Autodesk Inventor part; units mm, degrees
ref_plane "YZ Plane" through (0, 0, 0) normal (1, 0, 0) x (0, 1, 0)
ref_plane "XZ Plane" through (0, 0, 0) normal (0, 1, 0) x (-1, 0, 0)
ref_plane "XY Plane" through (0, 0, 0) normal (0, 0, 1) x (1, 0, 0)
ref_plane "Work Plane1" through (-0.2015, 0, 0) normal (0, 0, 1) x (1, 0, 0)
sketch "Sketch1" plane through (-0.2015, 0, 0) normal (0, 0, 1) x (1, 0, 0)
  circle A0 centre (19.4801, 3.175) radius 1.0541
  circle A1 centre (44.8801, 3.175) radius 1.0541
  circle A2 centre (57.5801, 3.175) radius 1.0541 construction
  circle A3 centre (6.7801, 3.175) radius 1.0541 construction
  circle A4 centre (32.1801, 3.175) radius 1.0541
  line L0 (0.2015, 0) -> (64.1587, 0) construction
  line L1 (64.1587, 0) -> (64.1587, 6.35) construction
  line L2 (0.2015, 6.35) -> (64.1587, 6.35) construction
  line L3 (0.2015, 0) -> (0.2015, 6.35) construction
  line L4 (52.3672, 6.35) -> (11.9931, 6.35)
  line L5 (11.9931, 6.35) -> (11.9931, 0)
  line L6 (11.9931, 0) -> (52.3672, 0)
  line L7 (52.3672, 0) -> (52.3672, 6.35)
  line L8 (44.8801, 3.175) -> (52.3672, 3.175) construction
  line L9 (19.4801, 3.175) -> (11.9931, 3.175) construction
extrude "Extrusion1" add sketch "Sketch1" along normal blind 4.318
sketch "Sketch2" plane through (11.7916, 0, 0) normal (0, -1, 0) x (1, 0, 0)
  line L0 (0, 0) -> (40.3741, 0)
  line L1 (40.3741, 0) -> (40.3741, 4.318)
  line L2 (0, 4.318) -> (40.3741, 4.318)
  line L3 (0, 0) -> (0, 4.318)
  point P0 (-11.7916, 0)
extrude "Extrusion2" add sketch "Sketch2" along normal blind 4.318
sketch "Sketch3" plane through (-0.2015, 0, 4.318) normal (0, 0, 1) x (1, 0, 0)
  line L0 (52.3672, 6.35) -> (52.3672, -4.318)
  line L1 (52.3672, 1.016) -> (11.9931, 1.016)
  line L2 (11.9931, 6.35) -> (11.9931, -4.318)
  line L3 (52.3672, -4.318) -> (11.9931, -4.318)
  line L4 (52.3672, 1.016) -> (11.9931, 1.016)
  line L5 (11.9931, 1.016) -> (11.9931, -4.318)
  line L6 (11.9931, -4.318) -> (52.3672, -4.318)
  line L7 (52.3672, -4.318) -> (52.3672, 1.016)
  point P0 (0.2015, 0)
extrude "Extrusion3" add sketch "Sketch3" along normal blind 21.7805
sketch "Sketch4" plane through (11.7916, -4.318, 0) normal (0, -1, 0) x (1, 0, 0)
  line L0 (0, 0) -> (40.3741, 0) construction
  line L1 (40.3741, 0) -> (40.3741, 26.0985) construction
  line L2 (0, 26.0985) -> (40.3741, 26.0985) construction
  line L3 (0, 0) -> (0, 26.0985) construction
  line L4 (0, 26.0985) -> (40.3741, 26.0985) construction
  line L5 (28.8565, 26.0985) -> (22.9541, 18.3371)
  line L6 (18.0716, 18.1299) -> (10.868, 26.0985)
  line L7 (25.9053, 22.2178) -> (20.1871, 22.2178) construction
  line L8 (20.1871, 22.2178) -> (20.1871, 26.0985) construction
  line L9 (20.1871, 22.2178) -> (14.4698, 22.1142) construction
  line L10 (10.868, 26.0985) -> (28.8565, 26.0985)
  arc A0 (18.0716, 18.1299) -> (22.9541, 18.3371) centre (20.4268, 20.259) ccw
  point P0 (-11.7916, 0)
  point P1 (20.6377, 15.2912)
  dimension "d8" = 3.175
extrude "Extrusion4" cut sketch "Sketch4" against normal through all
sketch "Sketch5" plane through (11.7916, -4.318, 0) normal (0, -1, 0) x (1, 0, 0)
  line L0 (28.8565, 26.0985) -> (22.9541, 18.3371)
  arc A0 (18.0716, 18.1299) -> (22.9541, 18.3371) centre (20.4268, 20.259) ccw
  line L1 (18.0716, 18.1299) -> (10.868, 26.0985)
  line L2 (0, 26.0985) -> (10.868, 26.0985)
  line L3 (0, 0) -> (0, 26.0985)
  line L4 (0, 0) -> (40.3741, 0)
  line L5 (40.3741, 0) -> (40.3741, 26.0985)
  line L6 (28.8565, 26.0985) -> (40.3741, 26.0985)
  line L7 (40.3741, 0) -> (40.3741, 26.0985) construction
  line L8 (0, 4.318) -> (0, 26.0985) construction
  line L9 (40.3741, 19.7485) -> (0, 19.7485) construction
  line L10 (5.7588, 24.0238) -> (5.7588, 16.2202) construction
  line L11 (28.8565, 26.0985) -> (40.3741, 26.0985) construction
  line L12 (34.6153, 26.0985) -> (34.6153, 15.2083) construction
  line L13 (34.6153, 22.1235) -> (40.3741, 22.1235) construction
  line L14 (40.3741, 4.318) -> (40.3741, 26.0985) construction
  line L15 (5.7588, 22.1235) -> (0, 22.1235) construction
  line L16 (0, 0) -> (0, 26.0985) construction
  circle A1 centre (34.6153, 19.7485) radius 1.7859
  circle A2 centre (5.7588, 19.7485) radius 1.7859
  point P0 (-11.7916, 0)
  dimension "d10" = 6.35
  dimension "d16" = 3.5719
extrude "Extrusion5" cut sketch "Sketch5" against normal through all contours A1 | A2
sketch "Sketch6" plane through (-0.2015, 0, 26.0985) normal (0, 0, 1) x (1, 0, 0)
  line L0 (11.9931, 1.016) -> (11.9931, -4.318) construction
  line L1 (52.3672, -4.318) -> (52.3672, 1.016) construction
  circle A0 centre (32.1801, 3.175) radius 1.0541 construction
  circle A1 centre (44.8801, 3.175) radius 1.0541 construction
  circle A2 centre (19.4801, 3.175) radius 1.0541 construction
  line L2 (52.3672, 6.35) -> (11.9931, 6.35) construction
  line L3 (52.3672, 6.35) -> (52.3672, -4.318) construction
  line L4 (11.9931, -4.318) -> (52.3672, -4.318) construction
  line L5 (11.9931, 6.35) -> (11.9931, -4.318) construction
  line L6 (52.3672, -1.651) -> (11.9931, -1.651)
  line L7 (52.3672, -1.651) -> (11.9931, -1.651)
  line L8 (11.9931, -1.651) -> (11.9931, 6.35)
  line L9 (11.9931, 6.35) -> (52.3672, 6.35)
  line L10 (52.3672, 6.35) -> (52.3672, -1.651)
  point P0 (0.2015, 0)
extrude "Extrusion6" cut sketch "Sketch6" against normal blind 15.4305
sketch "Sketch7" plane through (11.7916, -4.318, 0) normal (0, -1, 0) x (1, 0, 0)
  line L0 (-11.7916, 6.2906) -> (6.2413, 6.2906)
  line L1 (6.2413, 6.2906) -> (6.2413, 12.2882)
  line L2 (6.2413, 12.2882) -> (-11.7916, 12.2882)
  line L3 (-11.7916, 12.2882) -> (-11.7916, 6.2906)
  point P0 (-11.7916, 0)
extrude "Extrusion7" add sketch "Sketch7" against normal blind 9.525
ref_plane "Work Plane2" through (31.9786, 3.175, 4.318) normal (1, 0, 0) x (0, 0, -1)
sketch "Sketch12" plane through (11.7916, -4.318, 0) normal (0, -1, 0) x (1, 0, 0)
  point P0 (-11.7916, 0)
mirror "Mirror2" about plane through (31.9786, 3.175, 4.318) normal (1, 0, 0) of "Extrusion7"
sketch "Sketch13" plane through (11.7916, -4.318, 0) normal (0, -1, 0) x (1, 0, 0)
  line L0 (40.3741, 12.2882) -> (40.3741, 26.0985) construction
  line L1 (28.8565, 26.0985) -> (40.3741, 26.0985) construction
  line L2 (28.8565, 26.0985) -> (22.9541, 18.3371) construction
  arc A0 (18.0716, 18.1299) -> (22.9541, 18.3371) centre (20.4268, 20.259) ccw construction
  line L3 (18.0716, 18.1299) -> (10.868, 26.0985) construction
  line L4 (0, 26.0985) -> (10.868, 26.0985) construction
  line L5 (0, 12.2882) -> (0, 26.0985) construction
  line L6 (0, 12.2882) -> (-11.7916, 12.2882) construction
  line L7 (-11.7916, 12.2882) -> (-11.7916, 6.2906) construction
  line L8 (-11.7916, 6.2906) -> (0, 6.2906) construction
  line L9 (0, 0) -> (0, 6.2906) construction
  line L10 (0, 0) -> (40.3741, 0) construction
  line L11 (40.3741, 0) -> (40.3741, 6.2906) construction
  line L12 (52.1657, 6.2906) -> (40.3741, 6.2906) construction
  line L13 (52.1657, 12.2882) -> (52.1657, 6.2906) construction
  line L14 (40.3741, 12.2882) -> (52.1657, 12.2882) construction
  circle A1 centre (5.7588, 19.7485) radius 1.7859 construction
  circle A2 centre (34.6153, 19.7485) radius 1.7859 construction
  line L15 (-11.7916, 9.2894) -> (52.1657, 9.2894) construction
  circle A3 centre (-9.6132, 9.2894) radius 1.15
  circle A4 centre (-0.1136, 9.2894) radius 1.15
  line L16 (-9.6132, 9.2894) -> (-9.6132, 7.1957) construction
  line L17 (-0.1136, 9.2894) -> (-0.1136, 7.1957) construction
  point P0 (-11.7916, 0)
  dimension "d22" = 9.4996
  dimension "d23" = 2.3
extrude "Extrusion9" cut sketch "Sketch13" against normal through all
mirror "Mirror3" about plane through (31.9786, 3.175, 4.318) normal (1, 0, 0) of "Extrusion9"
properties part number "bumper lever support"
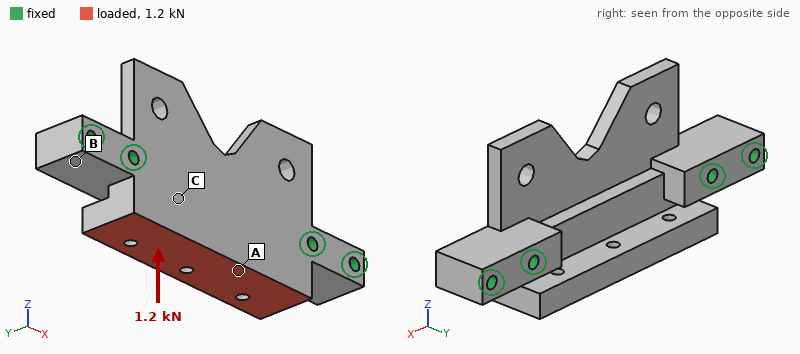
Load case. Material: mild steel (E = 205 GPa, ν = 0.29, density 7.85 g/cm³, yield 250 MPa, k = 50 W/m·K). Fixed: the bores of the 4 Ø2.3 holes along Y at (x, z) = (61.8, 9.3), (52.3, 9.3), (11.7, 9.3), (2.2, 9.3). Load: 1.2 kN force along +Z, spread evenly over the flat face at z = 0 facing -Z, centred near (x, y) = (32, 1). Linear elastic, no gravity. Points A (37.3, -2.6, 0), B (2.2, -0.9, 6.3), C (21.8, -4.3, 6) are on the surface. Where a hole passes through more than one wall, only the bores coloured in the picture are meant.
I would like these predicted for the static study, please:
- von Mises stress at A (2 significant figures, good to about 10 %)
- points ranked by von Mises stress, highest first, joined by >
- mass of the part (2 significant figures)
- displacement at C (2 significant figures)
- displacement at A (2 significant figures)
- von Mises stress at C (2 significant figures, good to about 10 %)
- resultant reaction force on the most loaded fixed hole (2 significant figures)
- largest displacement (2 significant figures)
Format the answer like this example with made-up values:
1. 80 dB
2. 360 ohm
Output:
1. 20 MPa
2. A > C > B
3. 48 g
4. 1.2 µm
5. 3.8 µm
6. 9.6 MPa
7. 680 N
8. 7.7 µm
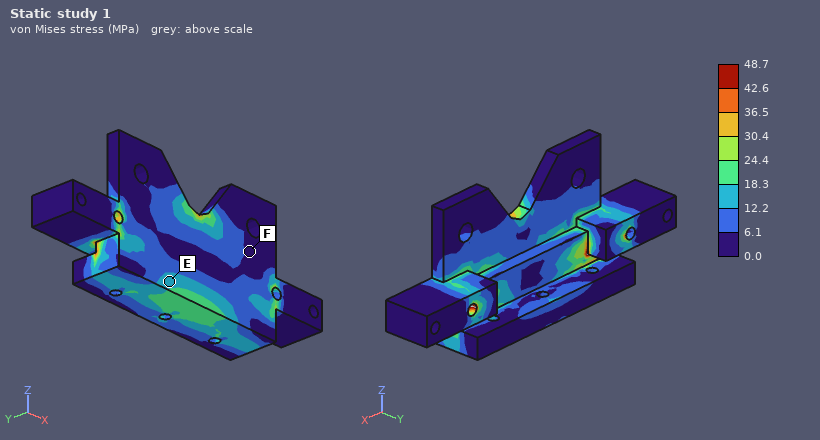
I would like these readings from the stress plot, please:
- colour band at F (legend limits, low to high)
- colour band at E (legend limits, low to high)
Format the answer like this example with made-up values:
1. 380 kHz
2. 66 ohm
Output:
1. 0.0 to 6.1 MPa
2. 12.2 to 18.3 MPa
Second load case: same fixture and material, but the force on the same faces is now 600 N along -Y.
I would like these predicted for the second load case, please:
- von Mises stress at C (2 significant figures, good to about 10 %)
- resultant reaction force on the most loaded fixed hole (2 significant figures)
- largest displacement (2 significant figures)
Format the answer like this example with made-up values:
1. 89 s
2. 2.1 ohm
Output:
1. 15 MPa
2. 310 N
3. 7.8 µm
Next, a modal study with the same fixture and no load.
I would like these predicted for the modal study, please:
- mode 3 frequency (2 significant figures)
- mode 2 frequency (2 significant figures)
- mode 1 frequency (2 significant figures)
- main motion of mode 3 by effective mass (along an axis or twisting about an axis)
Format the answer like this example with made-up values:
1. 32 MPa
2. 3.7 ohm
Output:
1. 15 kHz
2. 10 kHz
3. 8900 Hz
4. along Y
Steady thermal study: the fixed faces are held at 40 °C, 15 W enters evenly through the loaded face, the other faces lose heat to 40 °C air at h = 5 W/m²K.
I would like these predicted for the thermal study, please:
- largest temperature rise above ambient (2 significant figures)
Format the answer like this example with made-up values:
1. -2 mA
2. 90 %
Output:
1. 29 K
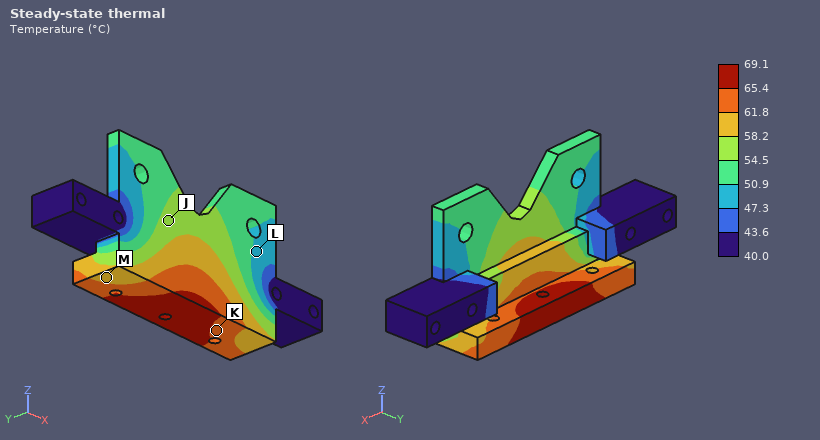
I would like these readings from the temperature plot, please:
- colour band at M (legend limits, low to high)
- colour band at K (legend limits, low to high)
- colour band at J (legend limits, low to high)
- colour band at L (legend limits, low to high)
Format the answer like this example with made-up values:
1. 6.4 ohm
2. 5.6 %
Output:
1. 58.2 to 61.8 °C
2. 61.8 to 65.4 °C
3. 54.5 to 58.2 °C
4. 47.3 to 50.9 °C
